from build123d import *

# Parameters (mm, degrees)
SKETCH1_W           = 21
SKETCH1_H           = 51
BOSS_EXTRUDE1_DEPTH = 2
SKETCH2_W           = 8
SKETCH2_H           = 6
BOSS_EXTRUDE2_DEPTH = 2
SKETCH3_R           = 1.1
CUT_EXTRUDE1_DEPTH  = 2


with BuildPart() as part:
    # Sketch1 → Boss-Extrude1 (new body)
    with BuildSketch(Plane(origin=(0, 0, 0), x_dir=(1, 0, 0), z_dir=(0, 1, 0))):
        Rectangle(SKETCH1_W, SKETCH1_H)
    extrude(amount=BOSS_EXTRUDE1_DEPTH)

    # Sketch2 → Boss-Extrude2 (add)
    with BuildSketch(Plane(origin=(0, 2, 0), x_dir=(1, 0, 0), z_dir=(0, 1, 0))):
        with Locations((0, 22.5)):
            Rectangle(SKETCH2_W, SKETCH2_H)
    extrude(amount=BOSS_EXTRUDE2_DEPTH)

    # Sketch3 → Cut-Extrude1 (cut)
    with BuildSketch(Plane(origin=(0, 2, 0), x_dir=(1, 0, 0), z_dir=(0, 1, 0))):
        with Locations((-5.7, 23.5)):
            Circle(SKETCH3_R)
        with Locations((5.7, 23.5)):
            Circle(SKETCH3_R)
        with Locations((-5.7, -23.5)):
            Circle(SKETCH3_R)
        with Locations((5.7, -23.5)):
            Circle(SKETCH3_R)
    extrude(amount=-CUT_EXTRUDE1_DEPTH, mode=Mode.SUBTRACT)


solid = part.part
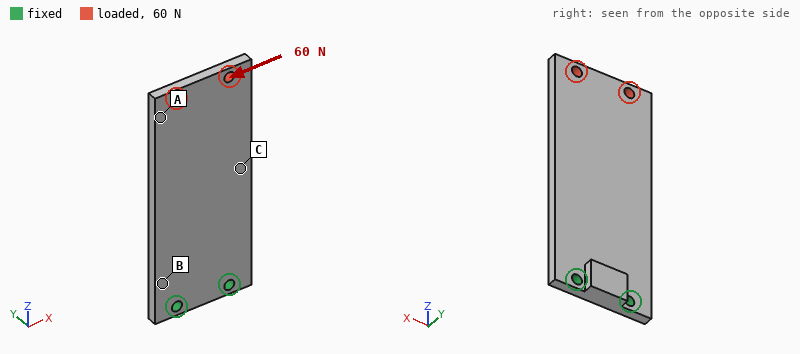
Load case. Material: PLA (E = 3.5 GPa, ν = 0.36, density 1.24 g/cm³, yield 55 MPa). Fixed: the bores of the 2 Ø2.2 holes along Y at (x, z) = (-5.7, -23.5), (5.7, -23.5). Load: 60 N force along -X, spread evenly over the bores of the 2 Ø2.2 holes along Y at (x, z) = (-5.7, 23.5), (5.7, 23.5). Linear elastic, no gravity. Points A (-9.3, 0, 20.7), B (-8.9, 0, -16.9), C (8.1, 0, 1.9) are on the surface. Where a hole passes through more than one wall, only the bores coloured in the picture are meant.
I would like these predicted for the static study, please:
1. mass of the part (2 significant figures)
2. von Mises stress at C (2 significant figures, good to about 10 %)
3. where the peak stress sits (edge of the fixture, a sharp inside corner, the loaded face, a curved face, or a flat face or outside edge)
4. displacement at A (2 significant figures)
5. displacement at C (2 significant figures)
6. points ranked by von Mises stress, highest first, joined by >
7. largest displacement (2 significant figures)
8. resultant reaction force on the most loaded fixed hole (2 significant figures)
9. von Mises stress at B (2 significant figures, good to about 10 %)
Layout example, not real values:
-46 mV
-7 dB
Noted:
2.7 g
7.0 MPa
edge of the fixture
0.52 mm
0.24 mm
B > C > A
0.59 mm
220 N
13 MPa
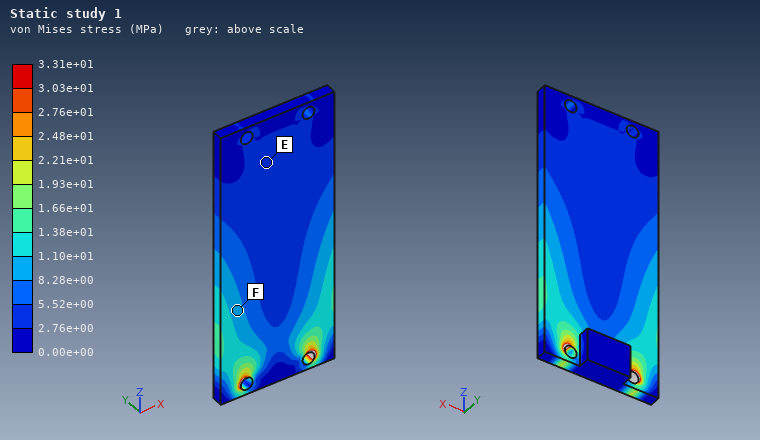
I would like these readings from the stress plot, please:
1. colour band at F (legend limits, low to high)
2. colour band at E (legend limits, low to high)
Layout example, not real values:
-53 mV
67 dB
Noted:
8.28e+00 to 1.10e+01 MPa
2.76e+00 to 5.52e+00 MPa
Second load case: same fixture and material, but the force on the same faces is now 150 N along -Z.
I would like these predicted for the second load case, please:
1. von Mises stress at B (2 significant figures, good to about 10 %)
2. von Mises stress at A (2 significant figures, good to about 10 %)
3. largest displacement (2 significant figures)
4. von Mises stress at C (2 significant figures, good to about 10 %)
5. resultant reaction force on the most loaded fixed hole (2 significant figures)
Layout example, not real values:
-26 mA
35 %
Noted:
3.3 MPa
3.0 MPa
66 µm
3.6 MPa
75 N
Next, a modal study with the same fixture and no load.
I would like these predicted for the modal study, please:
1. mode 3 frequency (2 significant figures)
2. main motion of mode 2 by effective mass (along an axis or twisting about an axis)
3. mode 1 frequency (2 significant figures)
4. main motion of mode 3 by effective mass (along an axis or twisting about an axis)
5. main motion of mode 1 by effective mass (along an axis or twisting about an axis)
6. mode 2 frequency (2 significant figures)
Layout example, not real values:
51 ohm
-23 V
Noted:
1500 Hz
twisting about Z
240 Hz
along Y
along Y
1100 Hz
